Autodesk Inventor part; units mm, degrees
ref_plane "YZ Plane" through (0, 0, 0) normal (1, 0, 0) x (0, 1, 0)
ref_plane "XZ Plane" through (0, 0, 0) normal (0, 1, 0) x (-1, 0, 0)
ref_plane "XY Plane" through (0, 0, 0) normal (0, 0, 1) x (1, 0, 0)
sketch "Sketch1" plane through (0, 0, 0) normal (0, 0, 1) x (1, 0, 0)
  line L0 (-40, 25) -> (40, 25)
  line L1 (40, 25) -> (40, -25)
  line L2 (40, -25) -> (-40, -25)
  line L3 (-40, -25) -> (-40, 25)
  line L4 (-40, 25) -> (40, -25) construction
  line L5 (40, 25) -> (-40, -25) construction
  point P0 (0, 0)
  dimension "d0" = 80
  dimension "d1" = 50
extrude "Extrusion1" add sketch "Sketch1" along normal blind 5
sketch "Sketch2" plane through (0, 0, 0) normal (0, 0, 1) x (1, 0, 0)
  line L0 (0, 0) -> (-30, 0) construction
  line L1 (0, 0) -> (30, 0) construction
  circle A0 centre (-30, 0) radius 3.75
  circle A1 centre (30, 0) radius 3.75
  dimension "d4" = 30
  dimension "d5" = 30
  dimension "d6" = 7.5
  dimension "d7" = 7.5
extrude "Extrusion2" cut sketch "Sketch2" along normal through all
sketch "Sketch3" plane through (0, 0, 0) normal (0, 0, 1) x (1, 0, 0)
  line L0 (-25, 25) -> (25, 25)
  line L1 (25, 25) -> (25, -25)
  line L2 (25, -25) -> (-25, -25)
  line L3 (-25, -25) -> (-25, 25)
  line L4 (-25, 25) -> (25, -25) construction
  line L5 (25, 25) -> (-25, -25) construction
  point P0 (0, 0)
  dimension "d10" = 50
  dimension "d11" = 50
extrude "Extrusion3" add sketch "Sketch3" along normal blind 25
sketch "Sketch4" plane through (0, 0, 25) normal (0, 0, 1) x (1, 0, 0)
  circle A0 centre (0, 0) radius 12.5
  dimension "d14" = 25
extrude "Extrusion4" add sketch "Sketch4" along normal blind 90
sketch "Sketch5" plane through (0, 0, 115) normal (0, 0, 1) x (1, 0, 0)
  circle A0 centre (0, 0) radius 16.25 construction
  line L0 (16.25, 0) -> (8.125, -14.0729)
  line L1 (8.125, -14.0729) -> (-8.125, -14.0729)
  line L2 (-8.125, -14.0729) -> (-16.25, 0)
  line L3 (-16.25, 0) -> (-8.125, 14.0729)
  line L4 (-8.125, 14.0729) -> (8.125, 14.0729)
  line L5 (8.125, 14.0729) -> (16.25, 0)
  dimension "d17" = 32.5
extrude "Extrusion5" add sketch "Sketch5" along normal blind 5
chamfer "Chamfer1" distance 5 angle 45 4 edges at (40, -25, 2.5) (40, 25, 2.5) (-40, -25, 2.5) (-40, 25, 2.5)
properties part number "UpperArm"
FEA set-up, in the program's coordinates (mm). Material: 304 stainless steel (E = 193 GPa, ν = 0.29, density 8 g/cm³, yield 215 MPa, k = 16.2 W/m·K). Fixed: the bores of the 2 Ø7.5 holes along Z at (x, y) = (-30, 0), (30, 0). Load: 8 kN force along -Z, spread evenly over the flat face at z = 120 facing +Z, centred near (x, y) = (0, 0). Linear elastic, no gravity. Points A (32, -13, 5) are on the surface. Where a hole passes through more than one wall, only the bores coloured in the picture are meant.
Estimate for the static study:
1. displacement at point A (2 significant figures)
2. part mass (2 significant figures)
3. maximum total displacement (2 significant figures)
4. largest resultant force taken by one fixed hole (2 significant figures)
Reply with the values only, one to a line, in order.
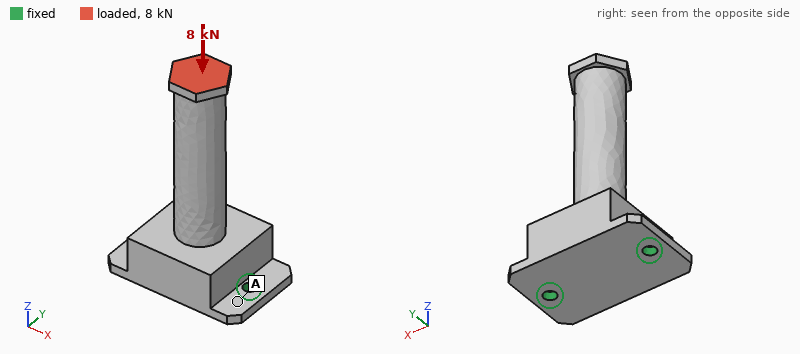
2.6 µm
940 g
16 µm
4.5 kN
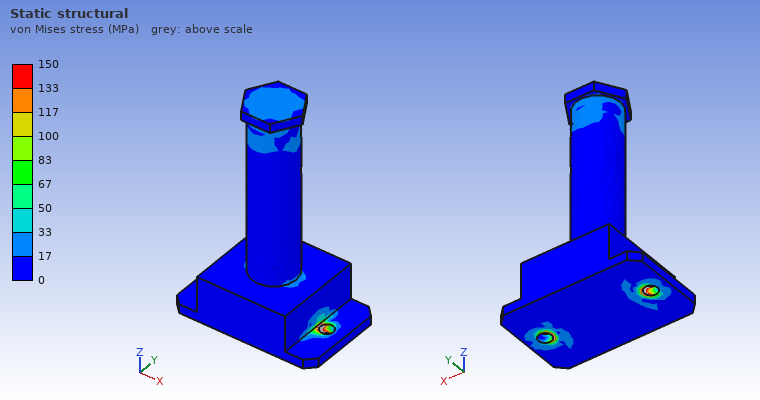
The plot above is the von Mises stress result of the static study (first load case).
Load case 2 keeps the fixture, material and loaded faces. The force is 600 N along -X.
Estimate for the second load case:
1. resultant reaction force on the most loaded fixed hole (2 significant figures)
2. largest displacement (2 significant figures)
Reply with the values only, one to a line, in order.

1.4 kN
66 µm
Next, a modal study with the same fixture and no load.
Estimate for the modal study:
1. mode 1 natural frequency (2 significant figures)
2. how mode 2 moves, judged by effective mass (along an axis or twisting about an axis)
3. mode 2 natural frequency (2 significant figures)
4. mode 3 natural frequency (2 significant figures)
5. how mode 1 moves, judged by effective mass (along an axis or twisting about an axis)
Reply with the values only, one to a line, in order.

660 Hz
along X
1500 Hz
4300 Hz
along Y
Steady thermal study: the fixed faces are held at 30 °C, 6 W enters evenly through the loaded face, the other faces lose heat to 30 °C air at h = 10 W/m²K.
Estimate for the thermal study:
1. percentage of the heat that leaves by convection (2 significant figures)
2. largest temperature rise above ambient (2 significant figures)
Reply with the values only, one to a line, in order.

53 %
60 K
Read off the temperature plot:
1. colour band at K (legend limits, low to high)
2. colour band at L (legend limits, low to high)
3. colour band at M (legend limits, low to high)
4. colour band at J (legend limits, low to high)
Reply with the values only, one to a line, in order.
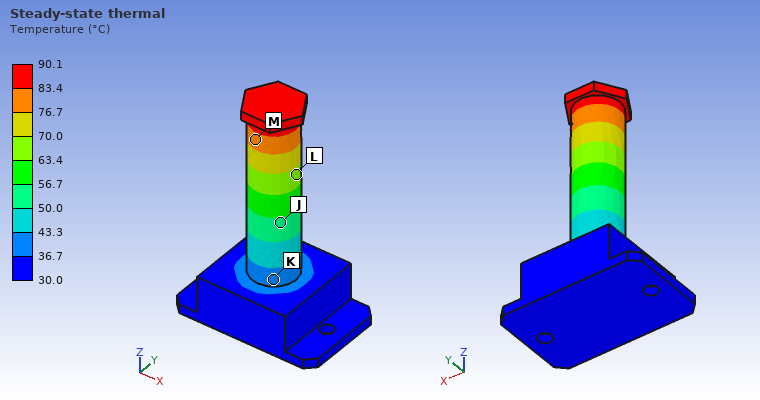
36.7 to 43.3 °C
63.4 to 70.0 °C
76.7 to 83.4 °C
50.0 to 56.7 °C
